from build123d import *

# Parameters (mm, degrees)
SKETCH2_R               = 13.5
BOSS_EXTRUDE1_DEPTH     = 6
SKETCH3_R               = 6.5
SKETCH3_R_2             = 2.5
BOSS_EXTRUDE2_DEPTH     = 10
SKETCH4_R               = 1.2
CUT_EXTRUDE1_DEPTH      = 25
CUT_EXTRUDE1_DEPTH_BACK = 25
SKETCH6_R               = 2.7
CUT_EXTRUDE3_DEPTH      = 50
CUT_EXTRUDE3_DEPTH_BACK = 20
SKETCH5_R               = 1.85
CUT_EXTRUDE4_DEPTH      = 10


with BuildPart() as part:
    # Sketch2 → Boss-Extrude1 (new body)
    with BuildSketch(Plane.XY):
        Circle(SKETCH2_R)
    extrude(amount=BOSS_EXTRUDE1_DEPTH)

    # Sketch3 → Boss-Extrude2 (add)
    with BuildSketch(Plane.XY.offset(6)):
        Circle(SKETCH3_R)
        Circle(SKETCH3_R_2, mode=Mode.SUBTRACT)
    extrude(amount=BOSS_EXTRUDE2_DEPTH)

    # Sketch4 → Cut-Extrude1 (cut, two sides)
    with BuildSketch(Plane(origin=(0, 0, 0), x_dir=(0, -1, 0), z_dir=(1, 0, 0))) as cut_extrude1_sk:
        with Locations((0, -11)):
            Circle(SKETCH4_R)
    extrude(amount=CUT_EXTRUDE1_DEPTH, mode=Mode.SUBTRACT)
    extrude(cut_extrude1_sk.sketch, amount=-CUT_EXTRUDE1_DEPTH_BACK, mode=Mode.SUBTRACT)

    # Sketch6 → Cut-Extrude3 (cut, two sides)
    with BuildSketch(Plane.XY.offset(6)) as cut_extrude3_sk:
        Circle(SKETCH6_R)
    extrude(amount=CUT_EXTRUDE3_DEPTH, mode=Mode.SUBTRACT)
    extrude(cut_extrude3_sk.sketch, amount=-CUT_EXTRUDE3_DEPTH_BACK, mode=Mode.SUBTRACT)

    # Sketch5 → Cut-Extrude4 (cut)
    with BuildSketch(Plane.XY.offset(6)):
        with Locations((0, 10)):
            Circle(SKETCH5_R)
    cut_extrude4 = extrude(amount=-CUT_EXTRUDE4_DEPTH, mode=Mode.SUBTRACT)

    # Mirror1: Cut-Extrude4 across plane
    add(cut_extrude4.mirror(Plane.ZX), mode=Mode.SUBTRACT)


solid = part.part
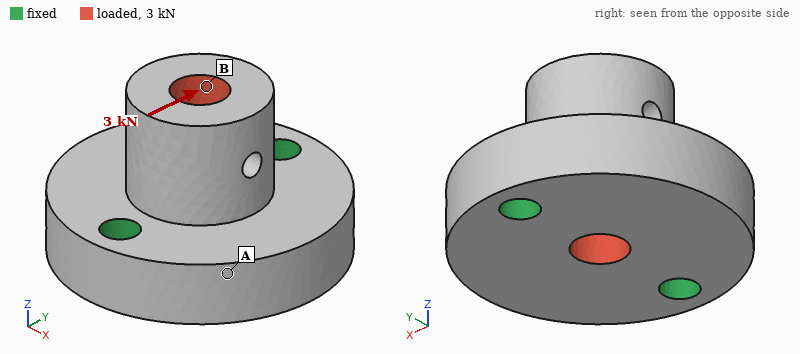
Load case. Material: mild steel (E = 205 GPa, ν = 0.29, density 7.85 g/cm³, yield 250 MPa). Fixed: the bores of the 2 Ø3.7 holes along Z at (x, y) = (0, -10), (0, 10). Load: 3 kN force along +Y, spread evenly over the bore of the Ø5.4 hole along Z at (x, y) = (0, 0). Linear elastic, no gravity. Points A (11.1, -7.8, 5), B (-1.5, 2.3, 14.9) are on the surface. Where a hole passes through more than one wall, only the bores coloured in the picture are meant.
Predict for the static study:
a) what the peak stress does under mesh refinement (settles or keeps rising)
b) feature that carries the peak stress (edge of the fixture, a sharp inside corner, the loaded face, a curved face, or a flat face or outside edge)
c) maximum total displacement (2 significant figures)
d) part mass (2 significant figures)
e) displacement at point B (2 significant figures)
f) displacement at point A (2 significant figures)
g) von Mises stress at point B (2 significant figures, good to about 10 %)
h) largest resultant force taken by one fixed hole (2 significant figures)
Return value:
keeps rising
a sharp inside corner
5.5 µm
33 g
4.9 µm
0.87 µm
19 MPa
1.7 kN
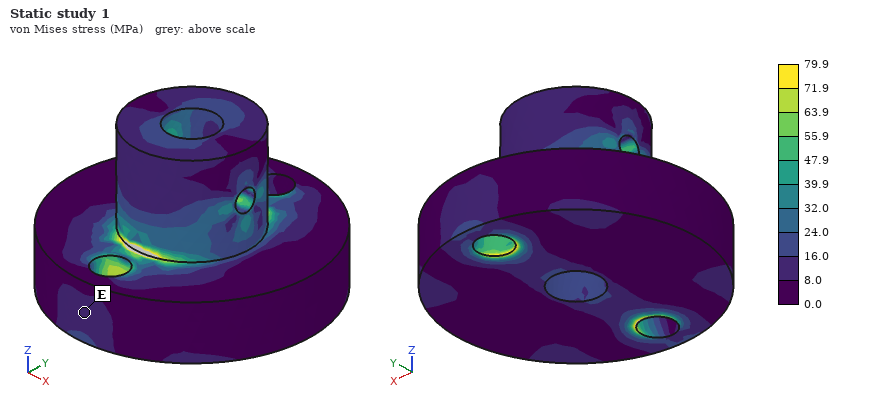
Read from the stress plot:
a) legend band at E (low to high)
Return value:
8.0 to 16.0 MPa
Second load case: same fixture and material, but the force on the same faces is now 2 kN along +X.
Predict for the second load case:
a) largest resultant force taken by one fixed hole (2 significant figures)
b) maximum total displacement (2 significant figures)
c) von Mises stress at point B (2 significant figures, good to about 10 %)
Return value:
1.0 kN
8.0 µm
16 MPa
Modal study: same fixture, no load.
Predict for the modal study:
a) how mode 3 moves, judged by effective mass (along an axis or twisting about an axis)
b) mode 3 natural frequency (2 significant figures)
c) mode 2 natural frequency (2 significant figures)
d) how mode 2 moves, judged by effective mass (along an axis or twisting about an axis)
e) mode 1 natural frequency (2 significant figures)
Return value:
along Y
37 kHz
31 kHz
along Z
19 kHz
